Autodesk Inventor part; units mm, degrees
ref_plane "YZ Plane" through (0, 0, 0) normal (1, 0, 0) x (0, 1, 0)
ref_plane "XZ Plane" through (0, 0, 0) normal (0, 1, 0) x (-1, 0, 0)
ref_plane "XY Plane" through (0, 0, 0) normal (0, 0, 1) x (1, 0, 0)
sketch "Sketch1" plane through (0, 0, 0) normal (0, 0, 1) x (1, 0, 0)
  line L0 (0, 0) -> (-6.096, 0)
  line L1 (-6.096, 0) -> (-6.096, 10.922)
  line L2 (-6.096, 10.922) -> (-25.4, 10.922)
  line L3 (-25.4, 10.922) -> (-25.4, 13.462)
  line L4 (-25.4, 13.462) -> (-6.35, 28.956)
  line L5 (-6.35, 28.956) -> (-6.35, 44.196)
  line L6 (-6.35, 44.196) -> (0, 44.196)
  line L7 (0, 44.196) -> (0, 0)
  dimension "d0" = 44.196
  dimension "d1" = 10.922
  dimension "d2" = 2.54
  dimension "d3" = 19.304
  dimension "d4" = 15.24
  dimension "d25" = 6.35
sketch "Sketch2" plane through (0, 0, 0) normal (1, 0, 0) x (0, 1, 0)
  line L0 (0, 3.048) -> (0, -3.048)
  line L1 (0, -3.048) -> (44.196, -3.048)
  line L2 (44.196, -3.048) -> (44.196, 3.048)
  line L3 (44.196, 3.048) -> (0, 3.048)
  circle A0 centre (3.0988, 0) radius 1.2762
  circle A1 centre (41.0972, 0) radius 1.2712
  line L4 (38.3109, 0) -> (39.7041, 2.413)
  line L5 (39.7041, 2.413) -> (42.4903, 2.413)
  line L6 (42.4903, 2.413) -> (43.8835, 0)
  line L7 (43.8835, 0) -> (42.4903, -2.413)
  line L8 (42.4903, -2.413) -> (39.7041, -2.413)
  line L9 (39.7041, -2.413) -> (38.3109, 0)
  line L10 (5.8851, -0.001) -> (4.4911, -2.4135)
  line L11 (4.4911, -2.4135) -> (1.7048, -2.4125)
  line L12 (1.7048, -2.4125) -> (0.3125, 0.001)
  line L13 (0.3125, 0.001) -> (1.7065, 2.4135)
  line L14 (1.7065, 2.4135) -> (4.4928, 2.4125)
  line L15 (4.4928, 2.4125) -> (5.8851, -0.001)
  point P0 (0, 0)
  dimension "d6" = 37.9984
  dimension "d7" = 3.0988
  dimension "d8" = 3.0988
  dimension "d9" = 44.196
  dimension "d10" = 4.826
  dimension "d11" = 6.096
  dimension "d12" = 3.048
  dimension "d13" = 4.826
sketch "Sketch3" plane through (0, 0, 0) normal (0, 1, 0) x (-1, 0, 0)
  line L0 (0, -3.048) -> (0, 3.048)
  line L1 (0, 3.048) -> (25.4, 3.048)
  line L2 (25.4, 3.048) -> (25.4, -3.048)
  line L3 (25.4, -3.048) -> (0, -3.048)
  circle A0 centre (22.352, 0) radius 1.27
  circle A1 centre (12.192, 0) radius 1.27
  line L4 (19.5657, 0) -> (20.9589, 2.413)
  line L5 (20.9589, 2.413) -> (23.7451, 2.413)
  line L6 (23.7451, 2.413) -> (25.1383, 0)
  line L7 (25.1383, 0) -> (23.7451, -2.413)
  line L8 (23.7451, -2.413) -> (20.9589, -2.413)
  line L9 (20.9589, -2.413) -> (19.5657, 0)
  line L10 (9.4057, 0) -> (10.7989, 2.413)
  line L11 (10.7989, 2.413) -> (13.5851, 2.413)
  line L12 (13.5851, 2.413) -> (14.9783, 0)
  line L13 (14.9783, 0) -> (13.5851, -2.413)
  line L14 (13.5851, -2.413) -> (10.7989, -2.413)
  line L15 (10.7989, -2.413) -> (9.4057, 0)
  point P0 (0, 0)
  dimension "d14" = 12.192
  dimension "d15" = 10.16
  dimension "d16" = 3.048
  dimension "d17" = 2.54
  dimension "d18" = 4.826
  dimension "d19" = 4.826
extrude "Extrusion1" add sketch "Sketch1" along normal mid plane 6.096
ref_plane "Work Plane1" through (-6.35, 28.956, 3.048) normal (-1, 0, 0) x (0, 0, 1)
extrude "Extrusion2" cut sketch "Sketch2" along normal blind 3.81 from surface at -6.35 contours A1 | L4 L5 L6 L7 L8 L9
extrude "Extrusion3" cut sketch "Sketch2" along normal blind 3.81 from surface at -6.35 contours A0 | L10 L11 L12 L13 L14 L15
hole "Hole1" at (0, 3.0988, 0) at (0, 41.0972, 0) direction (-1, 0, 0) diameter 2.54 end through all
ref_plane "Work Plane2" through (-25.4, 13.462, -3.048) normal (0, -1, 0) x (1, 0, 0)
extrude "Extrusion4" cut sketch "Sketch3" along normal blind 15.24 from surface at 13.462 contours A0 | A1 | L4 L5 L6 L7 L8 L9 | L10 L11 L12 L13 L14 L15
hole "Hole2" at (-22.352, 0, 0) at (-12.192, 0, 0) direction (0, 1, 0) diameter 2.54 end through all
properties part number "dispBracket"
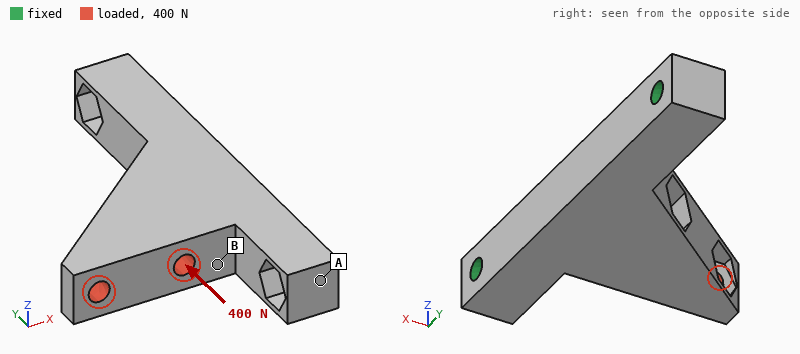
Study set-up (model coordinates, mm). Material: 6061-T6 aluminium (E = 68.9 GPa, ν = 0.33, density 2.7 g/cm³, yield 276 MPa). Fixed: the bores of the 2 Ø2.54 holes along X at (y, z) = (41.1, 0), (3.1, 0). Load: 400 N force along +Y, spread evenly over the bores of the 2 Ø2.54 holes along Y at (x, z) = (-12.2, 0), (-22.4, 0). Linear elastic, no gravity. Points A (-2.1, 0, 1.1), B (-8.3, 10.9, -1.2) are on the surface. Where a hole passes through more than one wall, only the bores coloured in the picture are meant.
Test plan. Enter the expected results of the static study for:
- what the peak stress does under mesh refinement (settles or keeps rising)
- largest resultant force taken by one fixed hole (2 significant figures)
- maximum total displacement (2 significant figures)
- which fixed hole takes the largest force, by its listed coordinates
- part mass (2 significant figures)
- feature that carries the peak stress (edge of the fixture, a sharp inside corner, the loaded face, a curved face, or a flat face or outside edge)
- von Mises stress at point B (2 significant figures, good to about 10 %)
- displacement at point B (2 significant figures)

keeps rising
320 N
36 µm
(41.1, 0)
6.5 g
edge of the fixture
32 MPa
5.5 µm
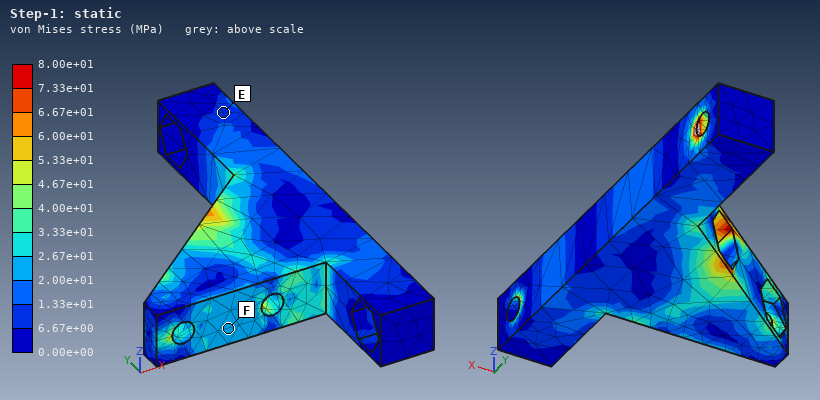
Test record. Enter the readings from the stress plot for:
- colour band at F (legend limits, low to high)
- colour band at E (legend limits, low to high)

2.00e+01 to 2.67e+01 MPa
6.67e+00 to 1.33e+01 MPa
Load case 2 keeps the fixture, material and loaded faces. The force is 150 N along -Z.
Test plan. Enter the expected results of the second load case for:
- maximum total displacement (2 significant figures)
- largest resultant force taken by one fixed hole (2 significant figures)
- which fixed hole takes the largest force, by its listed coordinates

0.13 mm
120 N
(3.1, 0)
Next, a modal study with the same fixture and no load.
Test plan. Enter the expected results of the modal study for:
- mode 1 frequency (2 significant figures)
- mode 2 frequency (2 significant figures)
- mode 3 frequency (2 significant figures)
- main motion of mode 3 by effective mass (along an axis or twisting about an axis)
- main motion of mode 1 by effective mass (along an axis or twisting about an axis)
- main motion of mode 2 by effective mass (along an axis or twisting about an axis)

5300 Hz
14 kHz
15 kHz
along Z
along Z
along X
